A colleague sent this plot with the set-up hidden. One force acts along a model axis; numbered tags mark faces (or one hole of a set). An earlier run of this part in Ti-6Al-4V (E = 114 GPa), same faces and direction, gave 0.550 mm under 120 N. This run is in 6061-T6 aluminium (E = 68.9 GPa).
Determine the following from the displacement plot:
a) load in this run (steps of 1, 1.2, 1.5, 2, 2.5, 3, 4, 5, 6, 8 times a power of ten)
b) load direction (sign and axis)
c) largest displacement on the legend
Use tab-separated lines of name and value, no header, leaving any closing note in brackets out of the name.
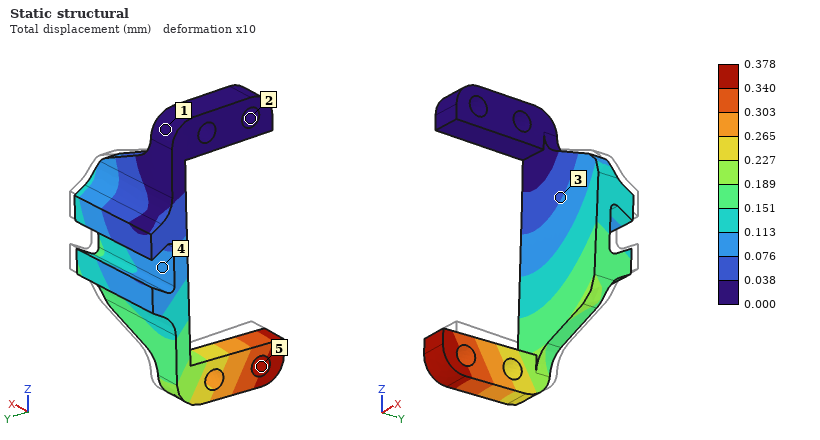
load in this run	50 N
load direction	-X
largest displacement on the legend	0.378 mm
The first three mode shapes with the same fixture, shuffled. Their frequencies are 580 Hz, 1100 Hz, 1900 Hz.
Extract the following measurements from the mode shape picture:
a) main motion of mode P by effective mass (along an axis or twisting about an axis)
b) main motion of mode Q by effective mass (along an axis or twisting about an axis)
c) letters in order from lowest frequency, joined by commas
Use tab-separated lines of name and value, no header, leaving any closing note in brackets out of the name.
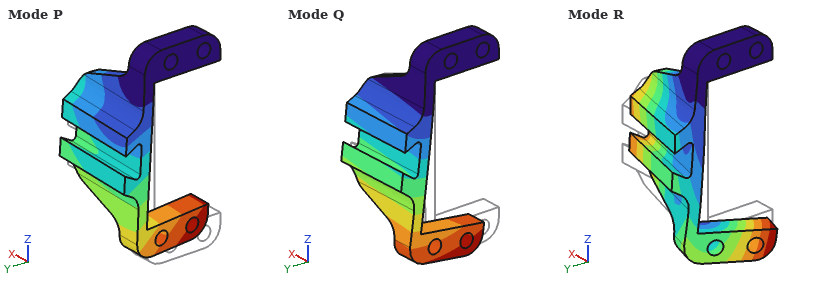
main motion of mode P by effective mass	along X
main motion of mode Q by effective mass	along Y
letters in order from lowest frequency, joined by commas	Q, P, R
